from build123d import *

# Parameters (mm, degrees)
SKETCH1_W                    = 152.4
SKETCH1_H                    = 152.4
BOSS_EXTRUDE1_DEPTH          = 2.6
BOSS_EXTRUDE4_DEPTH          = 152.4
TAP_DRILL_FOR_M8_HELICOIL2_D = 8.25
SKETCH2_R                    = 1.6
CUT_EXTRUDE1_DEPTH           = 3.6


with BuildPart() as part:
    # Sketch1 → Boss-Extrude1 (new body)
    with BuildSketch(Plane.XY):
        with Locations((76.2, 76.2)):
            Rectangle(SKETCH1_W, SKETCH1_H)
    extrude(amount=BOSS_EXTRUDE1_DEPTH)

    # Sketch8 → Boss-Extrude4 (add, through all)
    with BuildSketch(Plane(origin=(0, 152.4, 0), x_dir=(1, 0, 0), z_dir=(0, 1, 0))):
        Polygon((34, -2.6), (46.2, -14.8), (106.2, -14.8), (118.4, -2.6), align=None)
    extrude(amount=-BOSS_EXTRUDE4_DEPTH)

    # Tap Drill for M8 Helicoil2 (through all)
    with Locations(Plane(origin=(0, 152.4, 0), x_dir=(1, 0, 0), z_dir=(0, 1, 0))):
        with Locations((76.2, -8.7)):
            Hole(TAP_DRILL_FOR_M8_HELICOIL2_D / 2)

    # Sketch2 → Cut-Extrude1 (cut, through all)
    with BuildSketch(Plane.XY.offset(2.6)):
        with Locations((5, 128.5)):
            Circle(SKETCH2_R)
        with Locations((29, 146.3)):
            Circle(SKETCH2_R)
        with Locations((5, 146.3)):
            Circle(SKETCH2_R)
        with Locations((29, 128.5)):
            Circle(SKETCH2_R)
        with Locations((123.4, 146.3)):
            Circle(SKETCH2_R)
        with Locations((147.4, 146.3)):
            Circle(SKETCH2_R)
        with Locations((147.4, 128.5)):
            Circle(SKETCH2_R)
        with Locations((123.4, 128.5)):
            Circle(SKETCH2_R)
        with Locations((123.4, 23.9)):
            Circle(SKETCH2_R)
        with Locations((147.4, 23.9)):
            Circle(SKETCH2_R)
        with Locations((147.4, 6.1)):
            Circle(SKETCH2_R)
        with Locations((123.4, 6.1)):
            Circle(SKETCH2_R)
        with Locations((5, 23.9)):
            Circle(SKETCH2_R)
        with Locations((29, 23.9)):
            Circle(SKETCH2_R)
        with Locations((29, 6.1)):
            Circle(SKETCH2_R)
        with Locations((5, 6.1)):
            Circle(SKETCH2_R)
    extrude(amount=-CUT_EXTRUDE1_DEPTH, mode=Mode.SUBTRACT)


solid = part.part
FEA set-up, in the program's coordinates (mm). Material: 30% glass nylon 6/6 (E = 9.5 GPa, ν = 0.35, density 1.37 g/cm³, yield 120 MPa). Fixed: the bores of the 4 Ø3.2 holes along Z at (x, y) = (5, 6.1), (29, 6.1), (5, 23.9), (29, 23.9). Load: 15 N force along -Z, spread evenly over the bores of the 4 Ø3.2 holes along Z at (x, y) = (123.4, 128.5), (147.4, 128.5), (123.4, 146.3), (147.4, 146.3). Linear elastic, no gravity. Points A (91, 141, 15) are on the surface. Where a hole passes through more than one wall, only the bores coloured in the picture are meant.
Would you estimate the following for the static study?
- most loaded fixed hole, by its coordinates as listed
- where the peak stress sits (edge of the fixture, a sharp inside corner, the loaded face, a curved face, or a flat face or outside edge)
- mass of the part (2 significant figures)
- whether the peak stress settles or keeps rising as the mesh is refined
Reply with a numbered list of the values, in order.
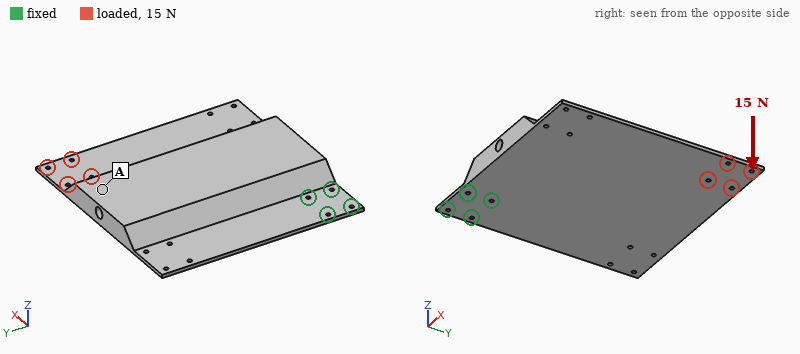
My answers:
1. (29, 23.9)
2. edge of the fixture
3. 260 g
4. keeps rising
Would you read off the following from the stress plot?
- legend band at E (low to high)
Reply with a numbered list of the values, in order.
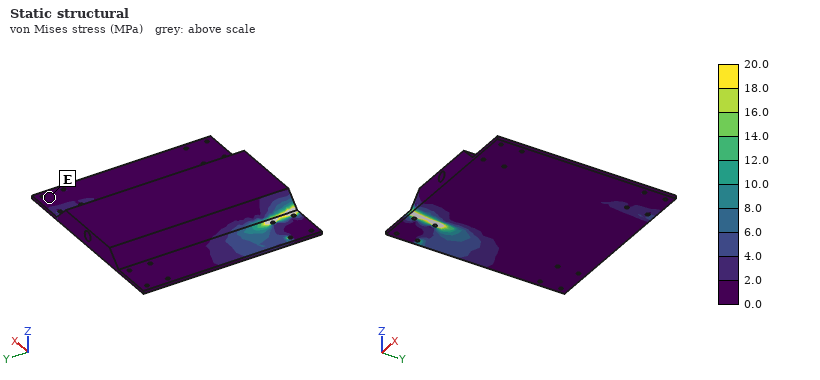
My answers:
1. 0.0 to 2.0 MPa
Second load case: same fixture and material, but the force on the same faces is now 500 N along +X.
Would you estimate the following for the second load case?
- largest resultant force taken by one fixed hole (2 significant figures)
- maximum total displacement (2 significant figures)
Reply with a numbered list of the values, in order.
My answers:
1. 1.4 kN
2. 1.4 mm
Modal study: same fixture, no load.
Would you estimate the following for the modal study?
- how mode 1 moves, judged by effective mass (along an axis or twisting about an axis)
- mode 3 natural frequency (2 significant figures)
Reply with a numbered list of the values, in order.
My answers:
1. along Z
2. 350 Hz
